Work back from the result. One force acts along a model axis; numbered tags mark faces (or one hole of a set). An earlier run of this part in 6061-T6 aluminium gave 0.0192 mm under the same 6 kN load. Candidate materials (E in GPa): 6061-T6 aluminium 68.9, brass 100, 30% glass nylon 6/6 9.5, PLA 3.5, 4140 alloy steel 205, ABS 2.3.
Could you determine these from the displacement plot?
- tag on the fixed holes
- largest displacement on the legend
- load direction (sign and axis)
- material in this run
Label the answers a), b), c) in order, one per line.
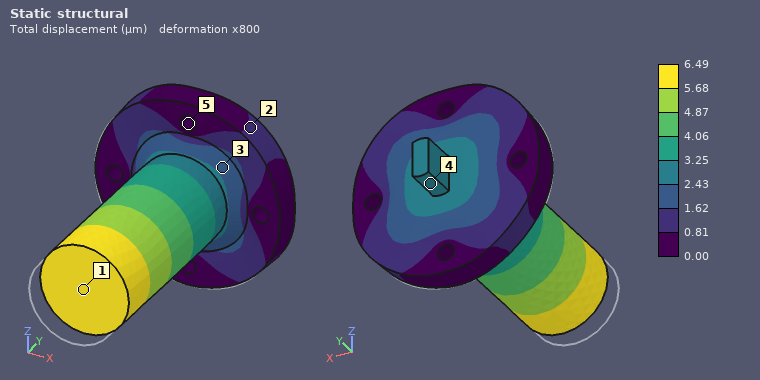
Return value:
a) 5
b) 6.49 µm
c) +Y
d) 4140 alloy steel
